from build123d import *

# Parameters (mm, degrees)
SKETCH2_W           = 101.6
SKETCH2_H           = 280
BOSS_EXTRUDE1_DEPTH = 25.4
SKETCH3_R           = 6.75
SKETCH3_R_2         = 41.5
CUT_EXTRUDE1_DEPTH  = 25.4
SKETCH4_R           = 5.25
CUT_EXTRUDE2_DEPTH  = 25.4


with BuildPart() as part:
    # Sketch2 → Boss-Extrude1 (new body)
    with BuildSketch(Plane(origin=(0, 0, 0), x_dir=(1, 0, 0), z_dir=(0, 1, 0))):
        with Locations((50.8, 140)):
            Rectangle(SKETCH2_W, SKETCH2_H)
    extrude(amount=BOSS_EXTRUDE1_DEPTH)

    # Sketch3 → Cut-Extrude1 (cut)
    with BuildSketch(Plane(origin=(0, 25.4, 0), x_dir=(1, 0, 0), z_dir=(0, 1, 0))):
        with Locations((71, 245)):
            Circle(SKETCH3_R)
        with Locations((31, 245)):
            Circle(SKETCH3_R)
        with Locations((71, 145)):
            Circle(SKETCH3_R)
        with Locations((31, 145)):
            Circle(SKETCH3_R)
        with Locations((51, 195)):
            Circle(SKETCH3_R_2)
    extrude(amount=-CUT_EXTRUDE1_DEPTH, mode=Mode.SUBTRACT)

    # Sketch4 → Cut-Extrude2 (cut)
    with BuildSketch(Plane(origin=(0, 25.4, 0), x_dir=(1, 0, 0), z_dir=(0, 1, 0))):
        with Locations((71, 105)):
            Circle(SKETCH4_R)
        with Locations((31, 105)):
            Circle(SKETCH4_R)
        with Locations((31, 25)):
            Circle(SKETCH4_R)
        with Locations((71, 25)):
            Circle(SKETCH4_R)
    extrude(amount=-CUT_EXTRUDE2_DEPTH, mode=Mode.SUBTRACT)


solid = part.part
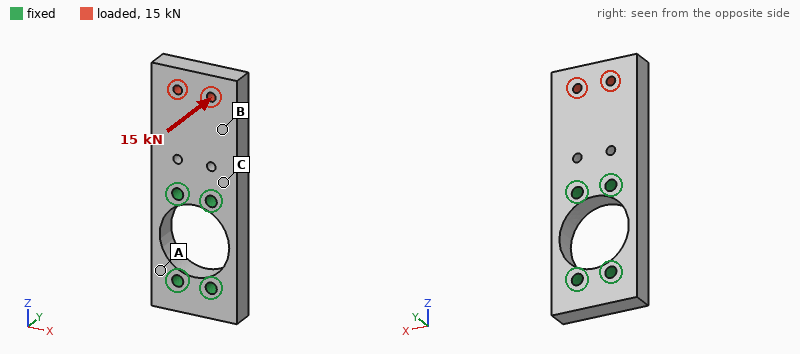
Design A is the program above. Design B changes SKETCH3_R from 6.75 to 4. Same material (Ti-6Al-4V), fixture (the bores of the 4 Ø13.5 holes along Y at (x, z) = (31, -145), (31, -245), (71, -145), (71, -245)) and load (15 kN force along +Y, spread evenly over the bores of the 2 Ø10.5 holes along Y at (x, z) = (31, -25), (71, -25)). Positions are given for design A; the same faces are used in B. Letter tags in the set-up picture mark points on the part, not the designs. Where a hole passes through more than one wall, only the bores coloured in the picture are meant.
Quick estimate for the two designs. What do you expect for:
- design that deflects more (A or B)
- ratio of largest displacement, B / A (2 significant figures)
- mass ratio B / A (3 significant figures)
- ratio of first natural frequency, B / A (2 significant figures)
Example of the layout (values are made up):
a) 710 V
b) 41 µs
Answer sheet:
a) B
b) 1.1
c) 1.02
d) 0.93
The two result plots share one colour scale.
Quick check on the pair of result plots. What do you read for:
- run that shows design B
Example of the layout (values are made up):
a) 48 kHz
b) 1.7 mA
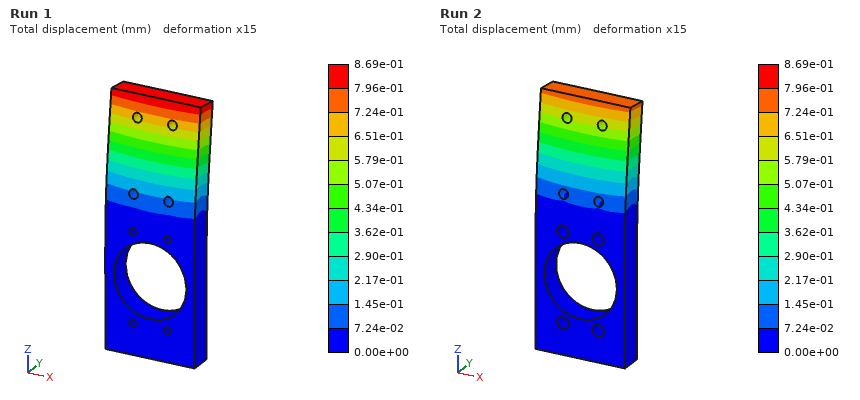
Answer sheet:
a) Run 1
